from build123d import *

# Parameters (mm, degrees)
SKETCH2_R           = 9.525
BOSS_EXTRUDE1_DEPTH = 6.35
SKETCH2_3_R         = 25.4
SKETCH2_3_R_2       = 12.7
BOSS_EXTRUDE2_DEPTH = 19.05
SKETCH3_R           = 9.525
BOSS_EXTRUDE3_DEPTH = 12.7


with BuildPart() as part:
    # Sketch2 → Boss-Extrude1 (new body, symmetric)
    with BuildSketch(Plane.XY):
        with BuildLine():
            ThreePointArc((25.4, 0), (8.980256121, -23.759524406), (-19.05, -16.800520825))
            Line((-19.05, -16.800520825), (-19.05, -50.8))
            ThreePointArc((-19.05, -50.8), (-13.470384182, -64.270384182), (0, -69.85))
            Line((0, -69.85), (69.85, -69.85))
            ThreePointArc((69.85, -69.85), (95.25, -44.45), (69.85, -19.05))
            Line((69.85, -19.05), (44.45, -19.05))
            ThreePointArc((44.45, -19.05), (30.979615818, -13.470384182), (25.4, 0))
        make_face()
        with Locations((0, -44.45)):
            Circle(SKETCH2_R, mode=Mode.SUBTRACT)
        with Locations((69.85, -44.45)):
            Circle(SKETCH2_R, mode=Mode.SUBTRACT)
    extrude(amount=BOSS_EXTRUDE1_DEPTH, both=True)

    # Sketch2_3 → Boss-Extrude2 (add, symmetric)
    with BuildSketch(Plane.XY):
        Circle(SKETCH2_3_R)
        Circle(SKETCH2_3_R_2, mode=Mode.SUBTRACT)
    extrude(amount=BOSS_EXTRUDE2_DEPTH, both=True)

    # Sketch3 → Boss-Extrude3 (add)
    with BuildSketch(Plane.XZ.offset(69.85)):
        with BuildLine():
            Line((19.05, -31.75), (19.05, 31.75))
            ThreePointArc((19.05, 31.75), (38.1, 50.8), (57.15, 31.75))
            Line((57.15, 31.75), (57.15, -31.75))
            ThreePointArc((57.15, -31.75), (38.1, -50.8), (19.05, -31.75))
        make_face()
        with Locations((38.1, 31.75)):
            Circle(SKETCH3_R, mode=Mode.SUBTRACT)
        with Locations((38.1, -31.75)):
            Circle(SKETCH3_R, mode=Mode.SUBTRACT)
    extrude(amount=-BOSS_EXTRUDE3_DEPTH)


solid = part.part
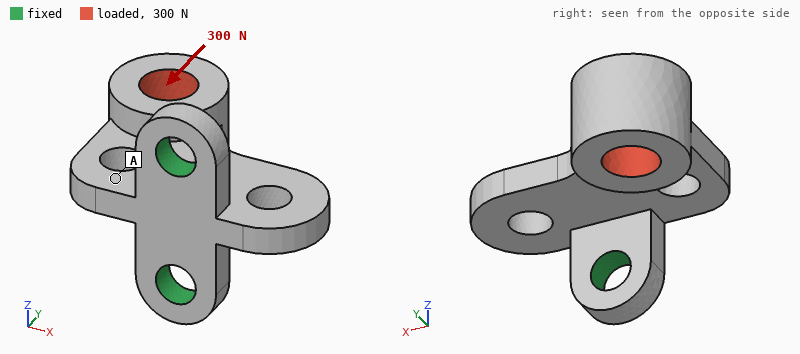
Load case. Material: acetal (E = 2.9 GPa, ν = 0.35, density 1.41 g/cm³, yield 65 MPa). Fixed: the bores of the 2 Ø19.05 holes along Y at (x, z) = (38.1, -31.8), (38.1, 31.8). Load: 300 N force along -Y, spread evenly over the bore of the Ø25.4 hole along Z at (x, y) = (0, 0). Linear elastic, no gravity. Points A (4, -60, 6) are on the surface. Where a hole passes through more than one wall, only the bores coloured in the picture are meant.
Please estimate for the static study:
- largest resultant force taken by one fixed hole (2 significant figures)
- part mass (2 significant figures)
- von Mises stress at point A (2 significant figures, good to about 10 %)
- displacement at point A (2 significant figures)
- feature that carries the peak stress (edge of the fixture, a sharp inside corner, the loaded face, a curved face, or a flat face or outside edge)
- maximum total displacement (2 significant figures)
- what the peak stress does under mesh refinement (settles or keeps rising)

160 N
210 g
0.80 MPa
0.16 mm
edge of the fixture
0.47 mm
keeps rising
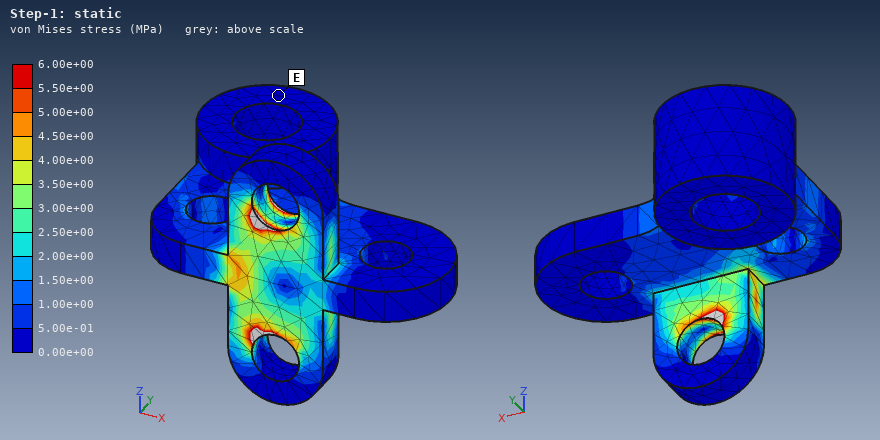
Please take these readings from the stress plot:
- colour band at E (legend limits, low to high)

0.00e+00 to 5.00e-01 MPa
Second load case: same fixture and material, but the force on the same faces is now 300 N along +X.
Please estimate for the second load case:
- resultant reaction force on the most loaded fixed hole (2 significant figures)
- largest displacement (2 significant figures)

150 N
0.78 mm
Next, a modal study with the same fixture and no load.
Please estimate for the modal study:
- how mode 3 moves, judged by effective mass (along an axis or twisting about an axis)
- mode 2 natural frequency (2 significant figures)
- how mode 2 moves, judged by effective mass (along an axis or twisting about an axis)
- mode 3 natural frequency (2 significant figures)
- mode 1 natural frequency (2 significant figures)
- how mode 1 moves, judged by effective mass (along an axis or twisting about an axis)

twisting about Y
320 Hz
along X
750 Hz
240 Hz
along Z
